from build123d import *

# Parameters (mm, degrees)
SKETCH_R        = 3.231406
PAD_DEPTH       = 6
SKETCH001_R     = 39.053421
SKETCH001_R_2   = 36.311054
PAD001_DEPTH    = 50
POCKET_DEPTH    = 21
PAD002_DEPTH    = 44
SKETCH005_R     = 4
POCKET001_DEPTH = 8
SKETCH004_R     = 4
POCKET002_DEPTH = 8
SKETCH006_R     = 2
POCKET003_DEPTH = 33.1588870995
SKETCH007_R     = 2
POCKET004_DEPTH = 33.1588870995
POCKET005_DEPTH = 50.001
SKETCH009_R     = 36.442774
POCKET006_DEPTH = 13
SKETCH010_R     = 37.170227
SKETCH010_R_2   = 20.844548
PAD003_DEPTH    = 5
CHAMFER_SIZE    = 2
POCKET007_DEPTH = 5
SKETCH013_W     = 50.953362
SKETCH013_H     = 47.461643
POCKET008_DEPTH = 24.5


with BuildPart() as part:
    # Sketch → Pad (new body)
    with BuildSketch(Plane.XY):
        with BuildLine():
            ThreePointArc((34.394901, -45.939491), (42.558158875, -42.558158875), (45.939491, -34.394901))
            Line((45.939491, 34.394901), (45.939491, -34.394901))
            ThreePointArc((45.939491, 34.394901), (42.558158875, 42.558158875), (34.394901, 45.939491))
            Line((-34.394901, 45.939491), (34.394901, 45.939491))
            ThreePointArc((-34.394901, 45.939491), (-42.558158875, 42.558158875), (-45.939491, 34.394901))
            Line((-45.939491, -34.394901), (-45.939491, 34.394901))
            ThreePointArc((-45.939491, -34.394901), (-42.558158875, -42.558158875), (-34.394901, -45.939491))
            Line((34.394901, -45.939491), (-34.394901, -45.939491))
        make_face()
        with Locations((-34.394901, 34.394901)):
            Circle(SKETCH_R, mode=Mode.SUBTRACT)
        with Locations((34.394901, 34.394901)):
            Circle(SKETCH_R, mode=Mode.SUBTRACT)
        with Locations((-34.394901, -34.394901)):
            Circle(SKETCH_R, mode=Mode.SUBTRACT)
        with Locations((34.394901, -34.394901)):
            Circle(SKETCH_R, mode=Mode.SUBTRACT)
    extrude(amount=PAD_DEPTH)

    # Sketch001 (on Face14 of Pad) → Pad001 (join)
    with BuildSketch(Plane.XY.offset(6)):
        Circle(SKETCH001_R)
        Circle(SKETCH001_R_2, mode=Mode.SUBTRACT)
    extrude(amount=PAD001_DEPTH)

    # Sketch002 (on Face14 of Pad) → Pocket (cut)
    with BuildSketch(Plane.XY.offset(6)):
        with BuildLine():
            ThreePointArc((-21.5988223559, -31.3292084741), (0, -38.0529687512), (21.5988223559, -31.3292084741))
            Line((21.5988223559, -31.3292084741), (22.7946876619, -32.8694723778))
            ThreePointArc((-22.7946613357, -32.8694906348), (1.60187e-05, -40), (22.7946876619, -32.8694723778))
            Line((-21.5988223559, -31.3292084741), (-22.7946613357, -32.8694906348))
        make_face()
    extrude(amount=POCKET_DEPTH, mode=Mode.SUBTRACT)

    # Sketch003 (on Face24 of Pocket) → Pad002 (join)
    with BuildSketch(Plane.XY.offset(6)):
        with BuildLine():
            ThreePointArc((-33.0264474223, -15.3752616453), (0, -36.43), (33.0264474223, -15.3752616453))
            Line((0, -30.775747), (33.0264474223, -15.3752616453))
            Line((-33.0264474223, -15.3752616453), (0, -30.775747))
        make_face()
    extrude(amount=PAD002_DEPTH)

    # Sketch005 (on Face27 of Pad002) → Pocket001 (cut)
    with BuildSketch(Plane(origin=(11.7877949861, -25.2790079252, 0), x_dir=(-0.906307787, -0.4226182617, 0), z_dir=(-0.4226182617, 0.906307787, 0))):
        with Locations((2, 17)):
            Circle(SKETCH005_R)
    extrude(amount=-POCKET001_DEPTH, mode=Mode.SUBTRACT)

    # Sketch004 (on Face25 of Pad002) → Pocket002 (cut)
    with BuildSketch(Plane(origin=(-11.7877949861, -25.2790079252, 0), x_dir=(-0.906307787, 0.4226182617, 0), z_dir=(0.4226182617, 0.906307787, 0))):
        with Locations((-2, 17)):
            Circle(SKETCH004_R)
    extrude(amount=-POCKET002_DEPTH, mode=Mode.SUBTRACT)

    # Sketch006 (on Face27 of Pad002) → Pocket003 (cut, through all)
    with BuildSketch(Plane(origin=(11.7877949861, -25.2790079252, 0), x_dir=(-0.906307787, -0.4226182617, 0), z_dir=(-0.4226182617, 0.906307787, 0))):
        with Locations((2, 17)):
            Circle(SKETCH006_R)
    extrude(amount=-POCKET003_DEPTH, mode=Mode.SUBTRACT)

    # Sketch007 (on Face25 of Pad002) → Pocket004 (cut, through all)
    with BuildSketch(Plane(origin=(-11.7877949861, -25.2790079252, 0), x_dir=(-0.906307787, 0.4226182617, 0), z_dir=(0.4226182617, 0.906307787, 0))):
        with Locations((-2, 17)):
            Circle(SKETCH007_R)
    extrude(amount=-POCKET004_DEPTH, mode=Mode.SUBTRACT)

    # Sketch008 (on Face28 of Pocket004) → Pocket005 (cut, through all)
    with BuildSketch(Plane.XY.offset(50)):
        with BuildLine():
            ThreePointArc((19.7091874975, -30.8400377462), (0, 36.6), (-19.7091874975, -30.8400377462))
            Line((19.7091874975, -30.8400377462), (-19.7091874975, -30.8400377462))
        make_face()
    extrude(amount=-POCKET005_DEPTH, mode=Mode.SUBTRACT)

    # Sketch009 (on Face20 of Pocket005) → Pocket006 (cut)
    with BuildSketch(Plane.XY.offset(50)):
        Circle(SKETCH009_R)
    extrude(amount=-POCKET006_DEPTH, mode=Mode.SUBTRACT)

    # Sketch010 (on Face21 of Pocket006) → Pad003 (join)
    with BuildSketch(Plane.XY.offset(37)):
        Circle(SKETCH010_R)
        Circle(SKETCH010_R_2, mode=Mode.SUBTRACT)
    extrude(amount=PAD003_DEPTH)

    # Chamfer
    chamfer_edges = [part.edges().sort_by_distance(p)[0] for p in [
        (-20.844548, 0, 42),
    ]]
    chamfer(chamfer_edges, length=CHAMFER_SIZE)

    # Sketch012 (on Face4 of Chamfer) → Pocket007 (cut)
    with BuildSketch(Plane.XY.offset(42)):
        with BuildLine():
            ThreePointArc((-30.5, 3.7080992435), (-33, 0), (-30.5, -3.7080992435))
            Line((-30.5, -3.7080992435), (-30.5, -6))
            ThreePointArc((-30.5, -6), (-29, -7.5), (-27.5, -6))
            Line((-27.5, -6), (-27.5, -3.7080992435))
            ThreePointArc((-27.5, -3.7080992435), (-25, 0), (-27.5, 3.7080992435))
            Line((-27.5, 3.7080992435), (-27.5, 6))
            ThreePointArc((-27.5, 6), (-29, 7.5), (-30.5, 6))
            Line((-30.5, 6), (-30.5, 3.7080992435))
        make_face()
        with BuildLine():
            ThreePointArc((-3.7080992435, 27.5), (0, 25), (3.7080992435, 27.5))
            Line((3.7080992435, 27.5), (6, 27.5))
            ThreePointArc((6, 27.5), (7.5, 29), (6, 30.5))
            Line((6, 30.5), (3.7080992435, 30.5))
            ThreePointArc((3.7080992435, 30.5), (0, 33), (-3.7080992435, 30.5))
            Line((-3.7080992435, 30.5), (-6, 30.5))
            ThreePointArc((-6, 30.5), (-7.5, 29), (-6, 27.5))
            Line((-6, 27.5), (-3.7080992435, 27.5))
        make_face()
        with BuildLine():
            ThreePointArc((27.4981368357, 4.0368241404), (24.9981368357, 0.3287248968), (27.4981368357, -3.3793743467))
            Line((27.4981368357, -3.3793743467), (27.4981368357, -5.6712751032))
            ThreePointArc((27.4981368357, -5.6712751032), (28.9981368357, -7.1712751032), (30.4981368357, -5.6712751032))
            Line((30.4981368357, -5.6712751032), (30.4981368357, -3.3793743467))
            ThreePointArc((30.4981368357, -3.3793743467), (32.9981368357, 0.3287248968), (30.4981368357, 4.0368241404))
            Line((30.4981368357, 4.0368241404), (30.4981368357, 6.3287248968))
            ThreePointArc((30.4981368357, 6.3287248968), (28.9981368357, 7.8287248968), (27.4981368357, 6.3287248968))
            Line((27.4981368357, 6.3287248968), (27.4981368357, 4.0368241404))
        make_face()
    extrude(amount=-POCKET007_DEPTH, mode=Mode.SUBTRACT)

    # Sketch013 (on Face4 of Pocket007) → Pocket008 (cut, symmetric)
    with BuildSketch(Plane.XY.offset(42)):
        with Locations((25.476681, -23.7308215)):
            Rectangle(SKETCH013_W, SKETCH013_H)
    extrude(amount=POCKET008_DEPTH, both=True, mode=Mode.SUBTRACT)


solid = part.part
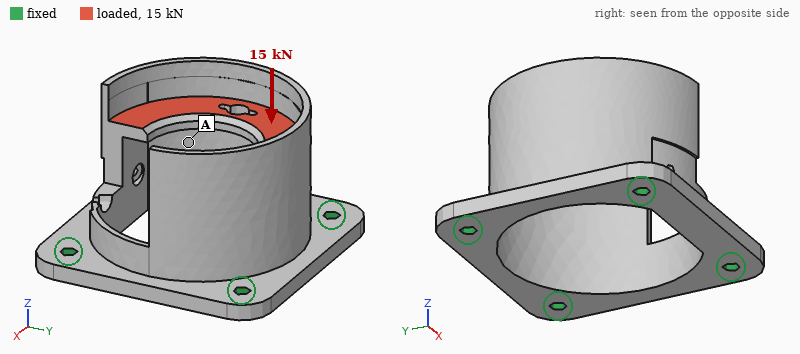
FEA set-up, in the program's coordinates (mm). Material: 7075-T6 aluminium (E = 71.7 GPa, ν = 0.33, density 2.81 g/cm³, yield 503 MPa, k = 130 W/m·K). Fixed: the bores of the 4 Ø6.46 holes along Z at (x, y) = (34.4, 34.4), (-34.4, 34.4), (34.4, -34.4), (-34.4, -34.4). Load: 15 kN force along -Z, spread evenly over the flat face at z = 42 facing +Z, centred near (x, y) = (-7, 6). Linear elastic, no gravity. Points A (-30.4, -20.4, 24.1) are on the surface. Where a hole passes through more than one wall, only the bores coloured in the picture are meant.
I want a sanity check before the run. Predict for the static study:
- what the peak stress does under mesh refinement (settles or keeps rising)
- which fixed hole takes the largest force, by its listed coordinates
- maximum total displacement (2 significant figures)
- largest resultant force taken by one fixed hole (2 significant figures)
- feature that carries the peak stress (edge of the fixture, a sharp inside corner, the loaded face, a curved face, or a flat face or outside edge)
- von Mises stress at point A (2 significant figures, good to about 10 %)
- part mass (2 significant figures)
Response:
keeps rising
(-34.4, 34.4)
0.42 mm
5.3 kN
edge of the fixture
49 MPa
170 g
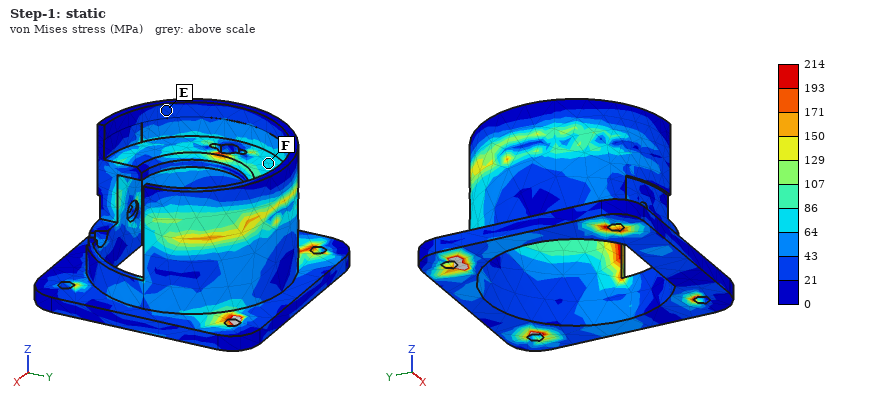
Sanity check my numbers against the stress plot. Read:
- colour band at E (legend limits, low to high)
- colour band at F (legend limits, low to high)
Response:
21 to 43 MPa
64 to 86 MPa
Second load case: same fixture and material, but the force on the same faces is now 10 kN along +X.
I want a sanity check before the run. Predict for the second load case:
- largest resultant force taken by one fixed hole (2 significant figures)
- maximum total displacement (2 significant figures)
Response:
5.8 kN
0.64 mm
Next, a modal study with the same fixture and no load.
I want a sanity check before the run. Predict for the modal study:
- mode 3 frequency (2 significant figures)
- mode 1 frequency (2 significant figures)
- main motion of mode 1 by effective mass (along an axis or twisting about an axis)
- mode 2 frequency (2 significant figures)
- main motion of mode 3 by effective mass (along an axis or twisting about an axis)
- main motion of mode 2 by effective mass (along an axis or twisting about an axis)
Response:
5000 Hz
3300 Hz
along X
3600 Hz
along X
along Y
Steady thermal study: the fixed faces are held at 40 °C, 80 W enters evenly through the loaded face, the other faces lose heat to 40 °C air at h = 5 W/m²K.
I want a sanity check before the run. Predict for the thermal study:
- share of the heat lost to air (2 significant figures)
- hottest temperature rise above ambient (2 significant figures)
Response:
6.2 %
63 K
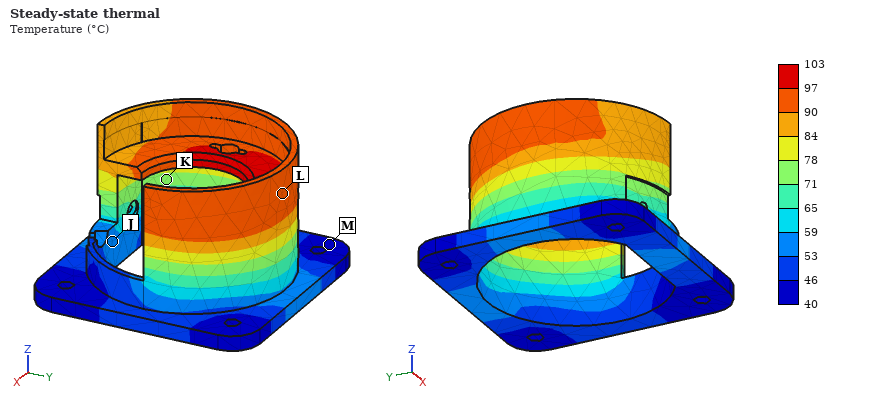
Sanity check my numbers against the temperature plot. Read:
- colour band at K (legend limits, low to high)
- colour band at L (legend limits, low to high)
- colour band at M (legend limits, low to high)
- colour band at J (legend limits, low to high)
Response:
71 to 78 °C
90 to 97 °C
40 to 46 °C
53 to 59 °C
